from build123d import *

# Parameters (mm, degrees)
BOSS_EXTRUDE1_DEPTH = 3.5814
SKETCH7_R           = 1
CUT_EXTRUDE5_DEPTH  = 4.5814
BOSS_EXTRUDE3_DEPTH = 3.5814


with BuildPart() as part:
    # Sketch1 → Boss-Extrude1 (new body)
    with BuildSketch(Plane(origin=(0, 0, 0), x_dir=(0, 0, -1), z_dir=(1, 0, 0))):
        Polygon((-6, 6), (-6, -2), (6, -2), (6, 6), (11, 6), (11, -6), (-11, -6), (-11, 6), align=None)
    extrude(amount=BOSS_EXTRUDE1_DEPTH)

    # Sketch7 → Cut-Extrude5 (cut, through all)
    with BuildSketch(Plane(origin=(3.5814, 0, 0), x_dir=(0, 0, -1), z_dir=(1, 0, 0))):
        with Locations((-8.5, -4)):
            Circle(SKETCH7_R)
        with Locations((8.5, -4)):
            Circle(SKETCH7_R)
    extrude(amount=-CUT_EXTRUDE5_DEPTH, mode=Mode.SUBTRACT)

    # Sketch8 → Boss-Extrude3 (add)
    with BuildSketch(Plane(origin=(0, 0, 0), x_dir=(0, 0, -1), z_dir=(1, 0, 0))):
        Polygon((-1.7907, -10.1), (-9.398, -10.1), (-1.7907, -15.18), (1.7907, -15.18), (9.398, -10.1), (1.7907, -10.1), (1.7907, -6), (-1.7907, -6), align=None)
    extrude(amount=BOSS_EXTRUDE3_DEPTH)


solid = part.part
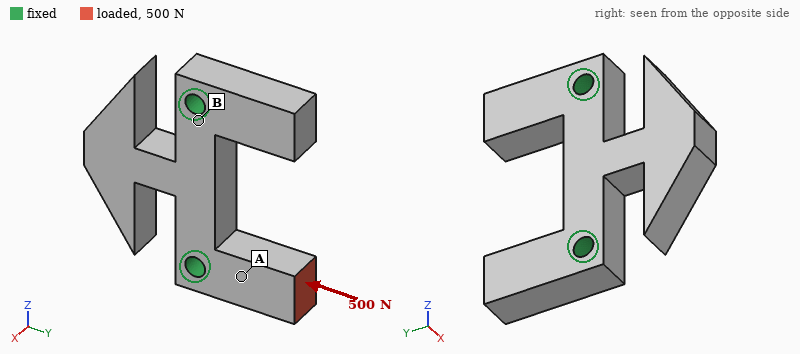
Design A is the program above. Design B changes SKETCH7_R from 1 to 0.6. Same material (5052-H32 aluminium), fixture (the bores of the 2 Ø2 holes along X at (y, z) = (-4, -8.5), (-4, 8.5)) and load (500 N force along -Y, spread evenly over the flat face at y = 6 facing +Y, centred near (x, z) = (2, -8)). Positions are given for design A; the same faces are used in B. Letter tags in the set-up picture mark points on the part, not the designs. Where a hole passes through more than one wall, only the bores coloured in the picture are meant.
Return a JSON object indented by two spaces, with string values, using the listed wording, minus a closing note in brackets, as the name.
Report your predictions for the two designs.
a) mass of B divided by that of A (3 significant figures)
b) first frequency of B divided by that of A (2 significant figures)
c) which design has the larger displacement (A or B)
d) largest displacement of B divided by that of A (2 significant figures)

{
  "mass of B divided by that of A": "1.02",
  "first frequency of B divided by that of A": "0.98",
  "which design has the larger displacement": "B",
  "largest displacement of B divided by that of A": "1.2"
}
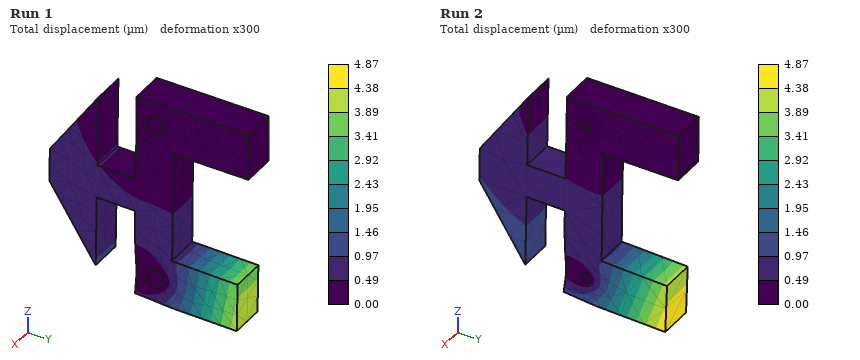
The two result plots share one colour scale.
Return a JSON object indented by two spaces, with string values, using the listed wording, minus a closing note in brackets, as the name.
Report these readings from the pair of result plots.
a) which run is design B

{
  "which run is design B": "Run 2"
}
